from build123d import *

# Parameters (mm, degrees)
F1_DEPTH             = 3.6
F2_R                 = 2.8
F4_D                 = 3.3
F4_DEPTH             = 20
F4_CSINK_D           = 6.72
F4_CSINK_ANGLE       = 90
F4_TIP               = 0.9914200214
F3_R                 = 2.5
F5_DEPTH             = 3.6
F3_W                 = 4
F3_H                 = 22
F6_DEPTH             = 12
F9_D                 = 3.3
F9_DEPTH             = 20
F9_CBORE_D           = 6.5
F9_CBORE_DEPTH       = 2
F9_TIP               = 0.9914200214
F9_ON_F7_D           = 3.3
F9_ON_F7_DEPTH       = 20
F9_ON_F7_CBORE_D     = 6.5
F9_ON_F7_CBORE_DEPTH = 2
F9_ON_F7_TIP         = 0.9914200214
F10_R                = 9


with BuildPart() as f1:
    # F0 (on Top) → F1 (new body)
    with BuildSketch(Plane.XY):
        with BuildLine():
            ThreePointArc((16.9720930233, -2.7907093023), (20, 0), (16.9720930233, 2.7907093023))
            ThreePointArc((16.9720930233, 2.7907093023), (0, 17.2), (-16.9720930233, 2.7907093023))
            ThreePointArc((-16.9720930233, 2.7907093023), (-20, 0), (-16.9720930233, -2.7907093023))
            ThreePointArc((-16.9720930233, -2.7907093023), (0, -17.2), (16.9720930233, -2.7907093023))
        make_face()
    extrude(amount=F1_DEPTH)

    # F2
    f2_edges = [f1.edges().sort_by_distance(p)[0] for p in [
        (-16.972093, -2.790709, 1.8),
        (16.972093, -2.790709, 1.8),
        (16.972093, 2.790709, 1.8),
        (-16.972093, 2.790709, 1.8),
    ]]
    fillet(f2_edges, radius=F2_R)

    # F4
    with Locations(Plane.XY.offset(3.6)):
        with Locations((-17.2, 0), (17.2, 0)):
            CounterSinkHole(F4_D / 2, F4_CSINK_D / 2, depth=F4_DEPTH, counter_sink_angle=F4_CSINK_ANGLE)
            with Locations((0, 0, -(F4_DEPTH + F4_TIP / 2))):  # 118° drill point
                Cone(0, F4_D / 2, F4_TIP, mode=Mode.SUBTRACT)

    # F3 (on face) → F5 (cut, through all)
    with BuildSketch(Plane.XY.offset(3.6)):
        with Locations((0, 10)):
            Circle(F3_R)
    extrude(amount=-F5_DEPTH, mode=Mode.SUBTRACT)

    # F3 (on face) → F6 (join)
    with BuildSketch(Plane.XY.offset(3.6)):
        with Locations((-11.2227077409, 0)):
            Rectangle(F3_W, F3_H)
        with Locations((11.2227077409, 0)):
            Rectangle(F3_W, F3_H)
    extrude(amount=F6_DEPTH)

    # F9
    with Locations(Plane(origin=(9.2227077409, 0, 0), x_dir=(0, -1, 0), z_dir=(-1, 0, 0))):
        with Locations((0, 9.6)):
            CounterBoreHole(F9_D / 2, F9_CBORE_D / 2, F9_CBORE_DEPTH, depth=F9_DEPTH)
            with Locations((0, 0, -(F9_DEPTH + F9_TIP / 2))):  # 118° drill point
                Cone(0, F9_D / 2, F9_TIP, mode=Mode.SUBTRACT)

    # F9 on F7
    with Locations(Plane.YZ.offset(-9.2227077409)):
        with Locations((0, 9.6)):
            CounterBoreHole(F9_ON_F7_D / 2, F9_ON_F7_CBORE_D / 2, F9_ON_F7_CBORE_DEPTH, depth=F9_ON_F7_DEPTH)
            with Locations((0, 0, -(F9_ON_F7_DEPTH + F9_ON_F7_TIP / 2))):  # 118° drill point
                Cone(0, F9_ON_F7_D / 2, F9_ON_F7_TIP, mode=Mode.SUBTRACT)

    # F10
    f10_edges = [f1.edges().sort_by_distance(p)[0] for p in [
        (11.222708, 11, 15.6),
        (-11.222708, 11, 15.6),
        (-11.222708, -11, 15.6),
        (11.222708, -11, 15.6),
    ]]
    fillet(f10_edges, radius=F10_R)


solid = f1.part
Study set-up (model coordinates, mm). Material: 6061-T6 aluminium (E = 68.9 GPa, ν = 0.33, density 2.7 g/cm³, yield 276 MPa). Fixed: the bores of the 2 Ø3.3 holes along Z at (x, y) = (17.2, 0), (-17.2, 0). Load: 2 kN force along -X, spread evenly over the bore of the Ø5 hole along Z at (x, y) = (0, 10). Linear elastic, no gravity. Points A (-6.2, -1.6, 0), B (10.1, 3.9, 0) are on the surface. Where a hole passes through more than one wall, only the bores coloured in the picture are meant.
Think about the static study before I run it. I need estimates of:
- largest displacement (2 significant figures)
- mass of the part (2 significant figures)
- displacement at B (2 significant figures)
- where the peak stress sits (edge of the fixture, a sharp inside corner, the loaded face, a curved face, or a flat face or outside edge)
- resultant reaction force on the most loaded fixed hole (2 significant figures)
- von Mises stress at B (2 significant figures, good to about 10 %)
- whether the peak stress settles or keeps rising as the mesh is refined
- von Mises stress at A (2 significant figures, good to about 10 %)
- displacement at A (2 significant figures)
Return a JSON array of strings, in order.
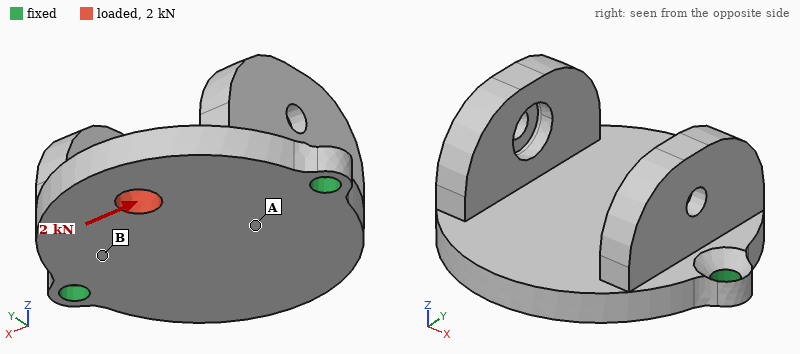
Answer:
["16 µm", "13 g", "6.1 µm", "edge of the fixture", "1.2 kN", "42 MPa", "keeps rising", "16 MPa", "4.2 µm"]
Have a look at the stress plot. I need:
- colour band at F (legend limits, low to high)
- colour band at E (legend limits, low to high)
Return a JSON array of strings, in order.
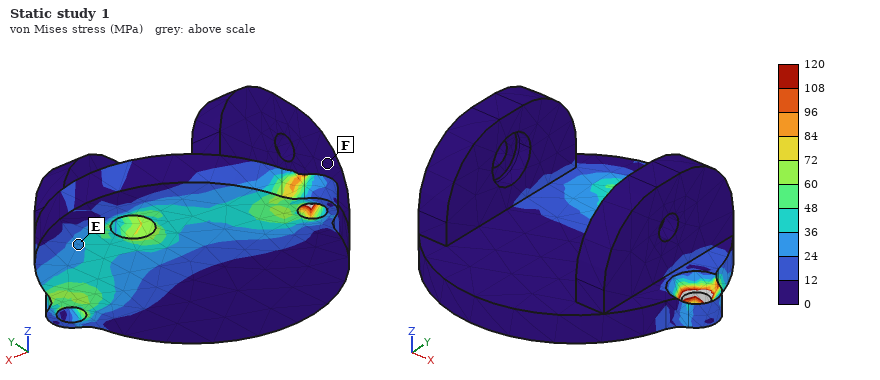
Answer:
["0 to 12 MPa", "24 to 36 MPa"]
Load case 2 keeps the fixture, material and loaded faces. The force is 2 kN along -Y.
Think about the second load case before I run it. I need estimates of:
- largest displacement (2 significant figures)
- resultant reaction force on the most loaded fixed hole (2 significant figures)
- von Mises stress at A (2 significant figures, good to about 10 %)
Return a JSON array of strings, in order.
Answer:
["27 µm", "1.0 kN", "17 MPa"]
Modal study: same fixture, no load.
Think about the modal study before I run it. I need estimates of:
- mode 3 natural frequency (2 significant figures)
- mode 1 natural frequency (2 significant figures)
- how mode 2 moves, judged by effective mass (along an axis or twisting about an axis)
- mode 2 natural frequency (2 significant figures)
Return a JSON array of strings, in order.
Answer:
["12 kHz", "4500 Hz", "along Z", "7500 Hz"]
